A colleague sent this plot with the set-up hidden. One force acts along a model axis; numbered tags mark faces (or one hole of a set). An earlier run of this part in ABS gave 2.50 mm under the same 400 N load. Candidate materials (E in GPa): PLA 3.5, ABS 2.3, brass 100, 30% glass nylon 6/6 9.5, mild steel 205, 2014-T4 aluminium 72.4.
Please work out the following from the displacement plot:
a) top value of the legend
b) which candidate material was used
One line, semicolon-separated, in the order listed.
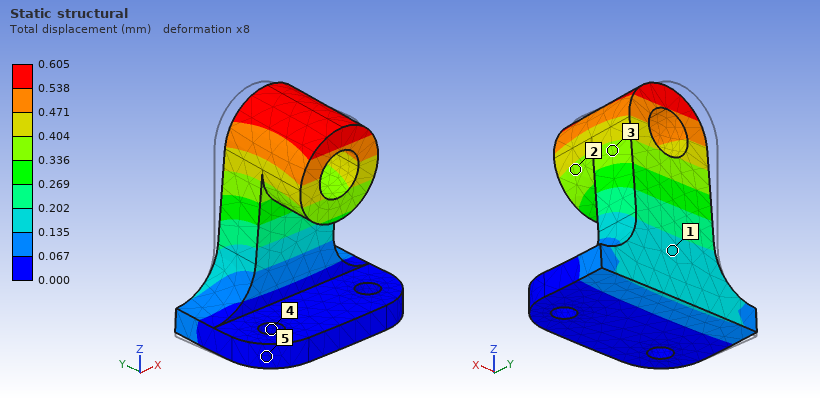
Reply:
0.605 mm; 30% glass nylon 6/6
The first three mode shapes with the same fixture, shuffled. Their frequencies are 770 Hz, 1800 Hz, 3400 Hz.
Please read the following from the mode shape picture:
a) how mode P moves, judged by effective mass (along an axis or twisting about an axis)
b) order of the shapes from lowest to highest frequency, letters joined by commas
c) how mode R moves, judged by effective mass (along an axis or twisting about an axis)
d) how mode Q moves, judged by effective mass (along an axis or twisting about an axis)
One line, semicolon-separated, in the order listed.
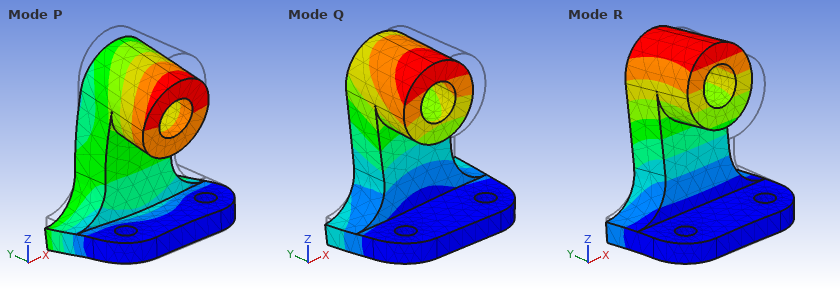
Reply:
along Z; R, Q, P; along Y; along X
